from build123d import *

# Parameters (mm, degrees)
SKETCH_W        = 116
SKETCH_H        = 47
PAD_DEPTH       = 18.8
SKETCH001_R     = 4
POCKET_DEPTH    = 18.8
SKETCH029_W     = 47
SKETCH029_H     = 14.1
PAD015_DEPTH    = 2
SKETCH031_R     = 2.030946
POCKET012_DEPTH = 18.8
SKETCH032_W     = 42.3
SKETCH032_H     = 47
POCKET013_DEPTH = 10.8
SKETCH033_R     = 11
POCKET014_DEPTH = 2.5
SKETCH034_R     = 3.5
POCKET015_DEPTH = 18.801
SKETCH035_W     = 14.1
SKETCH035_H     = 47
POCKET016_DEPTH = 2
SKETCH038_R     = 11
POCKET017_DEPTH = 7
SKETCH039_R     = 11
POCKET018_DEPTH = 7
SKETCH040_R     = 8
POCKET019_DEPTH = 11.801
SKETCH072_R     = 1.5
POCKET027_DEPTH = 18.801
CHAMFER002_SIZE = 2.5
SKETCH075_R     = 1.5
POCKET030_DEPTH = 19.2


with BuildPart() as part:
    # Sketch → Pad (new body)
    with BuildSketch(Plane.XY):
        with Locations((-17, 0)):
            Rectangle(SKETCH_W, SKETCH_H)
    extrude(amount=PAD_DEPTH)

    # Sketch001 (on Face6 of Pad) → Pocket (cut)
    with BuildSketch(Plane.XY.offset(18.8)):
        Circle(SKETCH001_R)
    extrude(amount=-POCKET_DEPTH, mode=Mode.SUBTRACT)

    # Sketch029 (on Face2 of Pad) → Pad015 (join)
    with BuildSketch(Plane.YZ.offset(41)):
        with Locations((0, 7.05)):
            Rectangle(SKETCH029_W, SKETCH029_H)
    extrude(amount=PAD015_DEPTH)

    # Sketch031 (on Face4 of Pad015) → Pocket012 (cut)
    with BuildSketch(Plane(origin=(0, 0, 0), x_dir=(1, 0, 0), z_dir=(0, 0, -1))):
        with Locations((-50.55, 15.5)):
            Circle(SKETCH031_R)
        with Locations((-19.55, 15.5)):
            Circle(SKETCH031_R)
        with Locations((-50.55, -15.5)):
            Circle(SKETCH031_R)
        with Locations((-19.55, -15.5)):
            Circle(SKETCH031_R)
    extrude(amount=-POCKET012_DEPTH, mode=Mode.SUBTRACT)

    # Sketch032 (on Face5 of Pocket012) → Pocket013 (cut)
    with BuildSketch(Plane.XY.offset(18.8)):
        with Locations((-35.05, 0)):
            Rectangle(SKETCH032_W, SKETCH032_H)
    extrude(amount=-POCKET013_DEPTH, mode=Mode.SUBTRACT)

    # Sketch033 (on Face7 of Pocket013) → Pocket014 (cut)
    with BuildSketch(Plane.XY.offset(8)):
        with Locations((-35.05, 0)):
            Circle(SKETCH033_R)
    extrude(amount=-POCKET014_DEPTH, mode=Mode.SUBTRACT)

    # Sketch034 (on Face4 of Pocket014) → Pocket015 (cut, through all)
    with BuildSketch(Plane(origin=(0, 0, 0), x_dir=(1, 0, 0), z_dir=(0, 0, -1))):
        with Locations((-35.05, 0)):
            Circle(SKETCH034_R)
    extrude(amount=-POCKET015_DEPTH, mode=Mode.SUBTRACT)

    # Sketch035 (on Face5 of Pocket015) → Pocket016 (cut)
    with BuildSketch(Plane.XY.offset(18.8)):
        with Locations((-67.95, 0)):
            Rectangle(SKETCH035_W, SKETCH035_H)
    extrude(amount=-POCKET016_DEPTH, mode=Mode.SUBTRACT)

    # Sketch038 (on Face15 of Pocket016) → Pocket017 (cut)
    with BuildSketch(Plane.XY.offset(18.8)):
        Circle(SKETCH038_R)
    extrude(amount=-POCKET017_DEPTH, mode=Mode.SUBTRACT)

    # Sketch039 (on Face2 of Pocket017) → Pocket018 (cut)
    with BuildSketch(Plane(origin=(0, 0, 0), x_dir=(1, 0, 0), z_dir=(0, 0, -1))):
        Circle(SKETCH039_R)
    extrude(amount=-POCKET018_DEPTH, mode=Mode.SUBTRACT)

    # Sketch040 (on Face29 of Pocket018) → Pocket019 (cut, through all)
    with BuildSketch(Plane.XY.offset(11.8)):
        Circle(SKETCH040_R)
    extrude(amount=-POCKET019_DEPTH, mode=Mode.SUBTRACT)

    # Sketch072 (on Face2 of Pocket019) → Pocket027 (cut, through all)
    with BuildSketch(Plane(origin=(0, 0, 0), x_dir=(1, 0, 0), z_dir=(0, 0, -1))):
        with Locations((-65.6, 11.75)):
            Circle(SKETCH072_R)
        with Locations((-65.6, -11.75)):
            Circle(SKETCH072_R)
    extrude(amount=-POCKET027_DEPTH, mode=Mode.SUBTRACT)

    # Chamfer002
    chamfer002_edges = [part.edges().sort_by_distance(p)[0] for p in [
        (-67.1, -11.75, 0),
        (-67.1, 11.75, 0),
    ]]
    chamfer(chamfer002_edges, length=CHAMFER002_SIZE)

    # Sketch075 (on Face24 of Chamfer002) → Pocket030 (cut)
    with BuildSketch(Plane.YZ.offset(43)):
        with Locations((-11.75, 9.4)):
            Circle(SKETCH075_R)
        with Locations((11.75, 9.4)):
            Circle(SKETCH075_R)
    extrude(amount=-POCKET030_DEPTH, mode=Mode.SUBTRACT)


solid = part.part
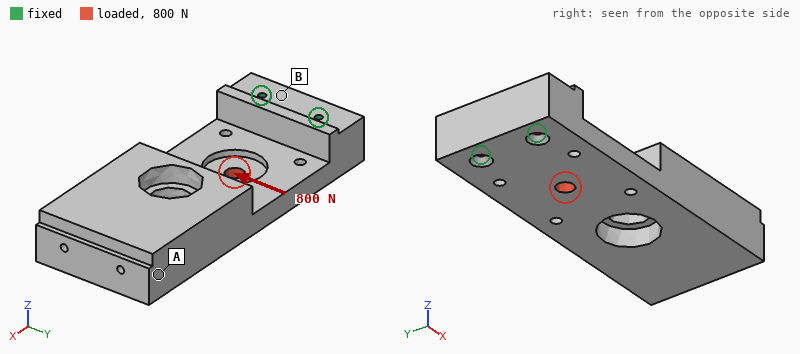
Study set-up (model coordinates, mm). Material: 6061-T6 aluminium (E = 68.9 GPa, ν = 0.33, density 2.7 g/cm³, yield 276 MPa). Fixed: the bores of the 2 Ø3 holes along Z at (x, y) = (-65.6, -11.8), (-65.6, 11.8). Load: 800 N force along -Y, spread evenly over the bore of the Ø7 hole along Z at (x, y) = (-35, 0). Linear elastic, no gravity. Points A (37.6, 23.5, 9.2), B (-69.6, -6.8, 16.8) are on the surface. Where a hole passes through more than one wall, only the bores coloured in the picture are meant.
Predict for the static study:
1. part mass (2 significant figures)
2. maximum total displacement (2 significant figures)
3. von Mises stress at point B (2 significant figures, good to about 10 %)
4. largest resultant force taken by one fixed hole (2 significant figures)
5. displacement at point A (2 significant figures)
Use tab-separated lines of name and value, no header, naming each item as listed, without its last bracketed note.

part mass	200 g
maximum total displacement	17 µm
von Mises stress at point B	2.7 MPa
largest resultant force taken by one fixed hole	1.1 kN
displacement at point A	16 µm
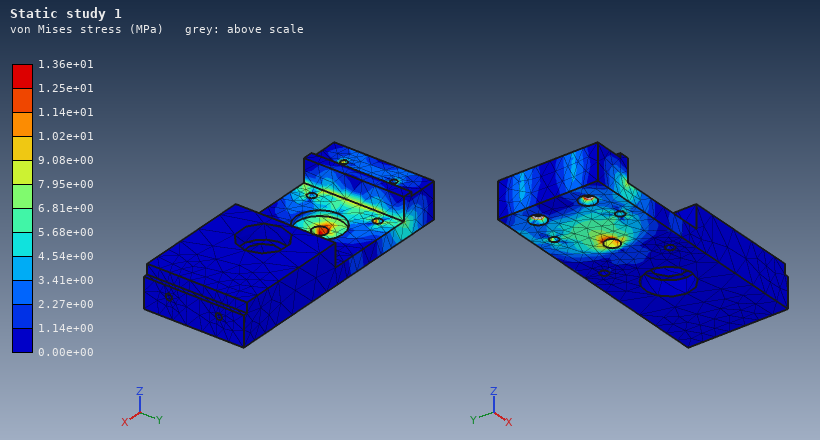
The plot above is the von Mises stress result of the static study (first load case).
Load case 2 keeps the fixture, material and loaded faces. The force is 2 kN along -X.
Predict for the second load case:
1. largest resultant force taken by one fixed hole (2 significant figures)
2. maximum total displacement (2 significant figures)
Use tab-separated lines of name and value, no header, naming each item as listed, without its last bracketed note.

largest resultant force taken by one fixed hole	1.0 kN
maximum total displacement	57 µm
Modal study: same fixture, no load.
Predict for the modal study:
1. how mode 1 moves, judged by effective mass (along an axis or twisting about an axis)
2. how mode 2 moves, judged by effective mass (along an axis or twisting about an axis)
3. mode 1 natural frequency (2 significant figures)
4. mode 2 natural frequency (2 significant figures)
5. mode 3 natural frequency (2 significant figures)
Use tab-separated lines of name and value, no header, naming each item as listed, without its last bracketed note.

how mode 1 moves, judged by effective mass	along Z
how mode 2 moves, judged by effective mass	along Y
mode 1 natural frequency	380 Hz
mode 2 natural frequency	1500 Hz
mode 3 natural frequency	2100 Hz
